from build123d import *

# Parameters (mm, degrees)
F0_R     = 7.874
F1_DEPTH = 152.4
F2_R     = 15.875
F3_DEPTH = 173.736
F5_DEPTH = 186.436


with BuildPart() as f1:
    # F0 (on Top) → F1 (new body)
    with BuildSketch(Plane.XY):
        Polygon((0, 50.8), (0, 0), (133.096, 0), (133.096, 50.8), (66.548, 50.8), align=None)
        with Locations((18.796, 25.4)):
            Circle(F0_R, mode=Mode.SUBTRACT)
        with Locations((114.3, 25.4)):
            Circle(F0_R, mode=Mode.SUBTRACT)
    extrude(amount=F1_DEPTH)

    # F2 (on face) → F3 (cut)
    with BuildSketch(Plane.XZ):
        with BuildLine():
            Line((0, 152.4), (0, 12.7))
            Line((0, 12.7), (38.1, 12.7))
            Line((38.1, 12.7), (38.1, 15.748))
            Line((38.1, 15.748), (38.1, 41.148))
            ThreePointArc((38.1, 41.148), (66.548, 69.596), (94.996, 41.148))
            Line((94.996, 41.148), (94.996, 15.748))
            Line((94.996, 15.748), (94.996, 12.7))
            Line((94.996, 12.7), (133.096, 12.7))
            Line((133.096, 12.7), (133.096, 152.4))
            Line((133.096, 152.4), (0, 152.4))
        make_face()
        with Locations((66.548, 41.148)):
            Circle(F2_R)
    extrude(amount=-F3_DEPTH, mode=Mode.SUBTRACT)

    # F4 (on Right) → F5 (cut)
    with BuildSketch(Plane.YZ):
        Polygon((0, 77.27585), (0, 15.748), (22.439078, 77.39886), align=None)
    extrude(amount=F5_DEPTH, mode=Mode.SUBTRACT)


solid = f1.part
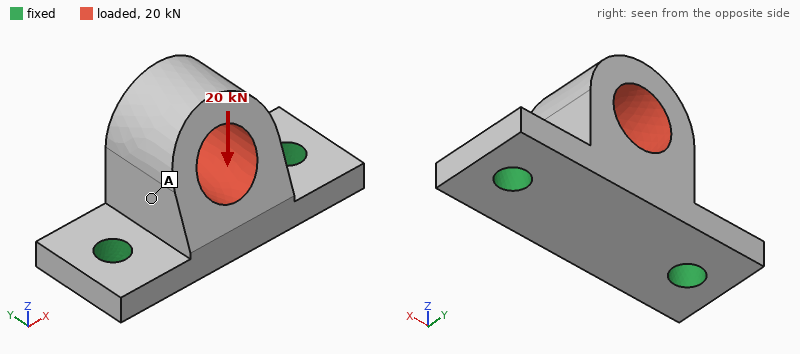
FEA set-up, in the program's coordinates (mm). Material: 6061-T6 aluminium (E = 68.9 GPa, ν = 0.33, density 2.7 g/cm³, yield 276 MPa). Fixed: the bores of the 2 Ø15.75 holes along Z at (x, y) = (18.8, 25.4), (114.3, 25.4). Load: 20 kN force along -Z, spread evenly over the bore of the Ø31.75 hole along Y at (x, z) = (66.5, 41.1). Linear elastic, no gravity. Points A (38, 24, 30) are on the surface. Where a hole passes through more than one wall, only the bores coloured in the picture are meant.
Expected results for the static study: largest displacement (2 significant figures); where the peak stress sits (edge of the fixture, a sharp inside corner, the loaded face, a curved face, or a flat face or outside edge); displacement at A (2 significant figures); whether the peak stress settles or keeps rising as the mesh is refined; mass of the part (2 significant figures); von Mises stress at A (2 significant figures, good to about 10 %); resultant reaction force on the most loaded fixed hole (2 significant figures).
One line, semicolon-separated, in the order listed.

82 µm; edge of the fixture; 39 µm; keeps rising; 460 g; 17 MPa; 11 kN
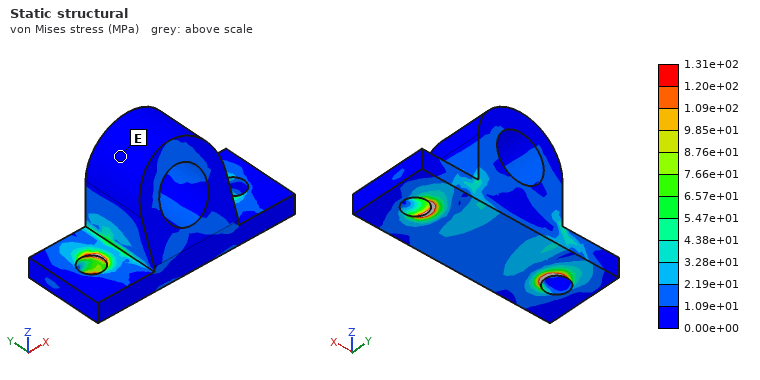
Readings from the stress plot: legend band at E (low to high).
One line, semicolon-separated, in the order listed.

0.00e+00 to 1.09e+01 MPa
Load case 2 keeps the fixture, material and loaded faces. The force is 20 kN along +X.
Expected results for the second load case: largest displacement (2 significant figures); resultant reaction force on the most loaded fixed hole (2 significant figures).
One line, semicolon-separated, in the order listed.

0.10 mm; 14 kN
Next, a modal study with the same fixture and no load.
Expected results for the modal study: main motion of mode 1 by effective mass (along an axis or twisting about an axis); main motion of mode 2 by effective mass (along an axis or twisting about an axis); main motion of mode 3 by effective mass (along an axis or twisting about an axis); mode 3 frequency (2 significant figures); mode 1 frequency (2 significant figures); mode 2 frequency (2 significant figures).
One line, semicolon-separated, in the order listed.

along Y; along X; along Z; 6200 Hz; 2700 Hz; 5700 Hz
